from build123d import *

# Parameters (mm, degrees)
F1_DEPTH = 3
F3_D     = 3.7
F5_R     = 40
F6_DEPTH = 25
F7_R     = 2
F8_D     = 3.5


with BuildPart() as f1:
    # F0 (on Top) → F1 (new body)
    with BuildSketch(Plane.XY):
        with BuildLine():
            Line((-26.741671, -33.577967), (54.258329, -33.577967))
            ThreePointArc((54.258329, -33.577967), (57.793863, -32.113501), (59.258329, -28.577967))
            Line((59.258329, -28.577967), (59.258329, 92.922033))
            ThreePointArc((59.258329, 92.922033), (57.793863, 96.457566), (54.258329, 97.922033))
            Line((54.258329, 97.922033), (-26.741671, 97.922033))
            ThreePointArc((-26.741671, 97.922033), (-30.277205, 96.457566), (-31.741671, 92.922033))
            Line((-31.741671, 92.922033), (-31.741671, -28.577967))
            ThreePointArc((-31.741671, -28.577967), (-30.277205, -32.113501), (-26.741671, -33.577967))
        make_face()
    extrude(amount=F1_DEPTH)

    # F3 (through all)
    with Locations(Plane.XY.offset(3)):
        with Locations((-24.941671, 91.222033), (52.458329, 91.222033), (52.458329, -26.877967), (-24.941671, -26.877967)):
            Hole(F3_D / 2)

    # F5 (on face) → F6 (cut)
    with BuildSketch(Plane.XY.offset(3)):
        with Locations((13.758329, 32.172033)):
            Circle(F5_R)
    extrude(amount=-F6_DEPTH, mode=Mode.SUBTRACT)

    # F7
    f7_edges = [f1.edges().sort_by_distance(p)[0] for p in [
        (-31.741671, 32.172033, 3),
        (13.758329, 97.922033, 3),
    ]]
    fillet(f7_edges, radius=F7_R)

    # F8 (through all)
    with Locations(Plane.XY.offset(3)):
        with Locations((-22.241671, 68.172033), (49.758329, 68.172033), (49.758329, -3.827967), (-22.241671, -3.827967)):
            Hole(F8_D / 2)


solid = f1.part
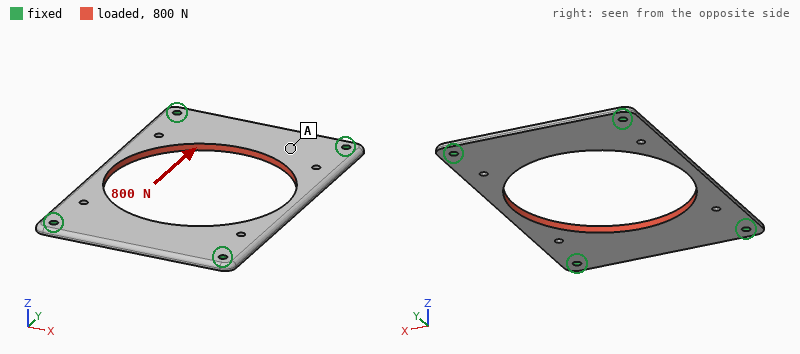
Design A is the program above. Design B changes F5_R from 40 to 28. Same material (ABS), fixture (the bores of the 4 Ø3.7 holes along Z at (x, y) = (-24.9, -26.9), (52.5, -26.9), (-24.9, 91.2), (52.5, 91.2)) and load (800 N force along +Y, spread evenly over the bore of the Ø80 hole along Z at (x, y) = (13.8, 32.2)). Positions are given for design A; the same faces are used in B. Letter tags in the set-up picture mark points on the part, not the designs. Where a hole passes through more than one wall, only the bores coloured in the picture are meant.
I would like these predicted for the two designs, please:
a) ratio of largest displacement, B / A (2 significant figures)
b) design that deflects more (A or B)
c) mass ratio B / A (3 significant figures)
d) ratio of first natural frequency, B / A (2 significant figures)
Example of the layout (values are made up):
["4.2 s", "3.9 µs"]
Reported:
["0.67", "A", "1.38", "0.74"]
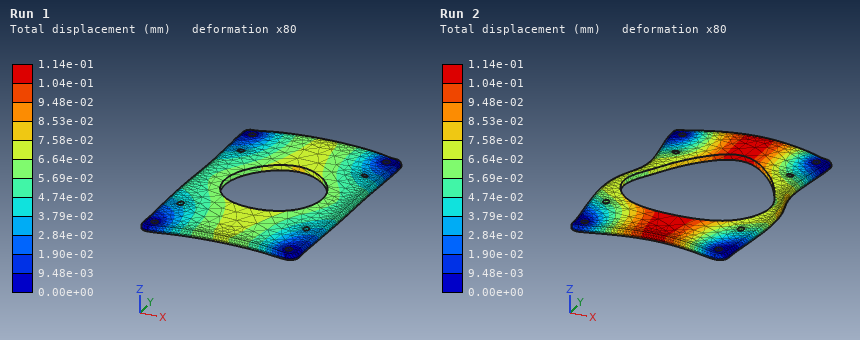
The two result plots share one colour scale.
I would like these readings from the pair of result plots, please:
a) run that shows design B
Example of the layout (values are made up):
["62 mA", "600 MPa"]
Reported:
["Run 1"]
